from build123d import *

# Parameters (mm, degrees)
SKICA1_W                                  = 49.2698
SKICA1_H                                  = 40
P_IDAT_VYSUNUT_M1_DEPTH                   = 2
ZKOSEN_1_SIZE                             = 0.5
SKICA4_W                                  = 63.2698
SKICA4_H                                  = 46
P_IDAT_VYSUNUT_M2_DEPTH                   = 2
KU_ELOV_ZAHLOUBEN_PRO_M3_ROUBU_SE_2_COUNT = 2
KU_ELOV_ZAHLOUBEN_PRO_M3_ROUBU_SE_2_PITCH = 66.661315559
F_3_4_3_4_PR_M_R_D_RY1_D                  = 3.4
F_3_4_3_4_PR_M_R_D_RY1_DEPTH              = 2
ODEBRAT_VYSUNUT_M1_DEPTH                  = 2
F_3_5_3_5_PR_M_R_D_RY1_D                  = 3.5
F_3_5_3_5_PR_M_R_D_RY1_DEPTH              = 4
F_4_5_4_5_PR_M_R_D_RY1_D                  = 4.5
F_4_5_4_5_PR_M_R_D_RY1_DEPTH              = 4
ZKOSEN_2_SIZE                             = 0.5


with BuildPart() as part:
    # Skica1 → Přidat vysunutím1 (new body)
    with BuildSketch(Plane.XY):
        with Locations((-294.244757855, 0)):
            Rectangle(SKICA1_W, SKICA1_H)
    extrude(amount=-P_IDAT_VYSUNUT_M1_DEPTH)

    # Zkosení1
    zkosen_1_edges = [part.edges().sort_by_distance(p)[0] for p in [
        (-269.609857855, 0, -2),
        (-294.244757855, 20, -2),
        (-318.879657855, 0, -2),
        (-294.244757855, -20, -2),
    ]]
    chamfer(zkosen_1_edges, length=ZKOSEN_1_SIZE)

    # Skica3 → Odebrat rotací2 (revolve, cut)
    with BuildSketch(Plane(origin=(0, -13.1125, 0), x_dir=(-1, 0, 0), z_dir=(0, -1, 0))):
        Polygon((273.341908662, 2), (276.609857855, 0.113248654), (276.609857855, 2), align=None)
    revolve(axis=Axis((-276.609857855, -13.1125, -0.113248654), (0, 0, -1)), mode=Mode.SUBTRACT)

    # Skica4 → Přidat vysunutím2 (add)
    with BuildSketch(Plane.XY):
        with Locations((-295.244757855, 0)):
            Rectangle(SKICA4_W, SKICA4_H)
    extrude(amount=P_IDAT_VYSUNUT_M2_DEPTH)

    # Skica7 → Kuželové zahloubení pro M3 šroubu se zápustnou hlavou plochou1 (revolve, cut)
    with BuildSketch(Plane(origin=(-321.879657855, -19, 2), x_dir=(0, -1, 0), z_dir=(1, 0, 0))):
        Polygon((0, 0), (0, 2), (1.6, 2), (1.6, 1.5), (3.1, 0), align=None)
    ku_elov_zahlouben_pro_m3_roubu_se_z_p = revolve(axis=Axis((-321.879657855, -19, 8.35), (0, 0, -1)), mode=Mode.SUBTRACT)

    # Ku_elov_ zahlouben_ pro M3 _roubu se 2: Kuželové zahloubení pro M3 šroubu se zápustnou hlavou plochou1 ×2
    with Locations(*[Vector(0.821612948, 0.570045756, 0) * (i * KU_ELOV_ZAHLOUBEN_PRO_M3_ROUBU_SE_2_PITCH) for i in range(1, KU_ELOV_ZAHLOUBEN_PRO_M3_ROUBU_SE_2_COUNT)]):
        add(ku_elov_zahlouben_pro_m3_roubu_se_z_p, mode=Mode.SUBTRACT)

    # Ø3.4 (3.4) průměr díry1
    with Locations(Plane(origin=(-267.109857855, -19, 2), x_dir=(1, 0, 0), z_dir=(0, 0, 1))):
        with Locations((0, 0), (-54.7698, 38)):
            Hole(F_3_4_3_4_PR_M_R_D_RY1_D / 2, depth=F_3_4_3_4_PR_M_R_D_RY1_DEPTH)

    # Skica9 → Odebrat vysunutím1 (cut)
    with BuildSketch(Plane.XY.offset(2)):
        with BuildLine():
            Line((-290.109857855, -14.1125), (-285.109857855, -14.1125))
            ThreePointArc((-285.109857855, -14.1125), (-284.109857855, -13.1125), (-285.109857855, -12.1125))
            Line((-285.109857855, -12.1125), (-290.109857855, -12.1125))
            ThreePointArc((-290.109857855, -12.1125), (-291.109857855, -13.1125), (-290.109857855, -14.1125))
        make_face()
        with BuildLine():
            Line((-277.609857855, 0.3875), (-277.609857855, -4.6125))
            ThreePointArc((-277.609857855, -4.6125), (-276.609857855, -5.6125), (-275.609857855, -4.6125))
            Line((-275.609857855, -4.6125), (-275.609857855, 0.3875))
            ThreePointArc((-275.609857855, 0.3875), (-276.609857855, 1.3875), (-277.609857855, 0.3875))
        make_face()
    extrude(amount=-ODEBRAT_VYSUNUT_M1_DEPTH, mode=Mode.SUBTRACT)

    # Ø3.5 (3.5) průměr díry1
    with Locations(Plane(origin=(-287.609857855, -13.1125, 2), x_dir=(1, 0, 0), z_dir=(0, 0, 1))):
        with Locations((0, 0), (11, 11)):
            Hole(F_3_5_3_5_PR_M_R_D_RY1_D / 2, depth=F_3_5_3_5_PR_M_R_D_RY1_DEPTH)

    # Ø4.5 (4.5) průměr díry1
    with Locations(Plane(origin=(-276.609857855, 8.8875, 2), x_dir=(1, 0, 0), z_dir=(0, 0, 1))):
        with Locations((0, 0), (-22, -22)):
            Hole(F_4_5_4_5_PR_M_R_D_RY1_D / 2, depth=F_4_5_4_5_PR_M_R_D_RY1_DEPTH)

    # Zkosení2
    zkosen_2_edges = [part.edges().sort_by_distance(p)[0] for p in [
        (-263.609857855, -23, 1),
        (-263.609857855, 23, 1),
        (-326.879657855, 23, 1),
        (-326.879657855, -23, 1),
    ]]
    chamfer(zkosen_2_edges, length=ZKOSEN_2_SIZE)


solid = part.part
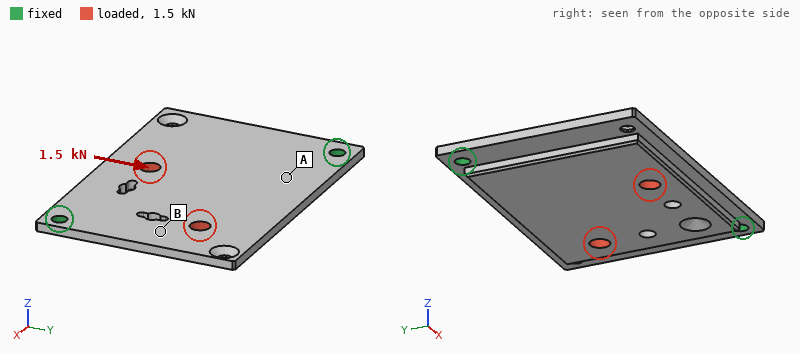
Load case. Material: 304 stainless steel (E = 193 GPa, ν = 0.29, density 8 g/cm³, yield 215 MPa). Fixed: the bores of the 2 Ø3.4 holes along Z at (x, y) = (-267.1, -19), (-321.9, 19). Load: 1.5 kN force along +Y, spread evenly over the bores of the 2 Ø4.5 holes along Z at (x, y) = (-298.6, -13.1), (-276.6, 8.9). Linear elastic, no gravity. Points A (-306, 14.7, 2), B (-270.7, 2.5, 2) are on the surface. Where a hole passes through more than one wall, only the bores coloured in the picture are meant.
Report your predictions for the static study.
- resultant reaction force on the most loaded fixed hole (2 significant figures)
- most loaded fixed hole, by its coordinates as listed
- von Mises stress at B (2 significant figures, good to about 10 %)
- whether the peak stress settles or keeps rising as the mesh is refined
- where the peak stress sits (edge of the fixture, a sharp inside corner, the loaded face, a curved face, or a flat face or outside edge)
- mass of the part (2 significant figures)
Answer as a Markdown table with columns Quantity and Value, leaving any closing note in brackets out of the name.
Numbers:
| Quantity | Value |
|---|---|
| resultant reaction force on the most loaded fixed hole | 900 N |
| most loaded fixed hole, by its coordinates as listed | (-267.1, -19) |
| von Mises stress at B | 19 MPa |
| whether the peak stress settles or keeps rising as the mesh is refined | keeps rising |
| where the peak stress sits | edge of the fixture |
| mass of the part | 75 g |
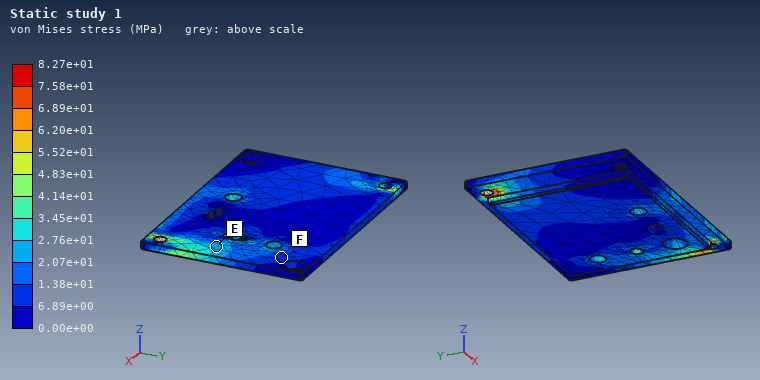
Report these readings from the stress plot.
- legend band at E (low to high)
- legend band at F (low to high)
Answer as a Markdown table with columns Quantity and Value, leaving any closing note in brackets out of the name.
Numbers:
| Quantity | Value |
|---|---|
| legend band at E | 2.07e+01 to 2.76e+01 MPa |
| legend band at F | 6.89e+00 to 1.38e+01 MPa |
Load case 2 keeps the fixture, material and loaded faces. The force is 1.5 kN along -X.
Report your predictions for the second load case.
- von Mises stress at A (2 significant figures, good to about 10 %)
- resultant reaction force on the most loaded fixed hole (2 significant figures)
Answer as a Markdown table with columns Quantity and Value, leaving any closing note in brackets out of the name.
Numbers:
| Quantity | Value |
|---|---|
| von Mises stress at A | 15 MPa |
| resultant reaction force on the most loaded fixed hole | 780 N |
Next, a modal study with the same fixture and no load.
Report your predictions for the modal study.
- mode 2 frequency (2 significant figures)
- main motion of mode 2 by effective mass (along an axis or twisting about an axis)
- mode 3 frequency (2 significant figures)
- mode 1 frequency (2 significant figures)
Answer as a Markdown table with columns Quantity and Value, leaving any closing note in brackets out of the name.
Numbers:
| Quantity | Value |
|---|---|
| mode 2 frequency | 2200 Hz |
| main motion of mode 2 by effective mass | along Z |
| mode 3 frequency | 5900 Hz |
| mode 1 frequency | 1400 Hz |
